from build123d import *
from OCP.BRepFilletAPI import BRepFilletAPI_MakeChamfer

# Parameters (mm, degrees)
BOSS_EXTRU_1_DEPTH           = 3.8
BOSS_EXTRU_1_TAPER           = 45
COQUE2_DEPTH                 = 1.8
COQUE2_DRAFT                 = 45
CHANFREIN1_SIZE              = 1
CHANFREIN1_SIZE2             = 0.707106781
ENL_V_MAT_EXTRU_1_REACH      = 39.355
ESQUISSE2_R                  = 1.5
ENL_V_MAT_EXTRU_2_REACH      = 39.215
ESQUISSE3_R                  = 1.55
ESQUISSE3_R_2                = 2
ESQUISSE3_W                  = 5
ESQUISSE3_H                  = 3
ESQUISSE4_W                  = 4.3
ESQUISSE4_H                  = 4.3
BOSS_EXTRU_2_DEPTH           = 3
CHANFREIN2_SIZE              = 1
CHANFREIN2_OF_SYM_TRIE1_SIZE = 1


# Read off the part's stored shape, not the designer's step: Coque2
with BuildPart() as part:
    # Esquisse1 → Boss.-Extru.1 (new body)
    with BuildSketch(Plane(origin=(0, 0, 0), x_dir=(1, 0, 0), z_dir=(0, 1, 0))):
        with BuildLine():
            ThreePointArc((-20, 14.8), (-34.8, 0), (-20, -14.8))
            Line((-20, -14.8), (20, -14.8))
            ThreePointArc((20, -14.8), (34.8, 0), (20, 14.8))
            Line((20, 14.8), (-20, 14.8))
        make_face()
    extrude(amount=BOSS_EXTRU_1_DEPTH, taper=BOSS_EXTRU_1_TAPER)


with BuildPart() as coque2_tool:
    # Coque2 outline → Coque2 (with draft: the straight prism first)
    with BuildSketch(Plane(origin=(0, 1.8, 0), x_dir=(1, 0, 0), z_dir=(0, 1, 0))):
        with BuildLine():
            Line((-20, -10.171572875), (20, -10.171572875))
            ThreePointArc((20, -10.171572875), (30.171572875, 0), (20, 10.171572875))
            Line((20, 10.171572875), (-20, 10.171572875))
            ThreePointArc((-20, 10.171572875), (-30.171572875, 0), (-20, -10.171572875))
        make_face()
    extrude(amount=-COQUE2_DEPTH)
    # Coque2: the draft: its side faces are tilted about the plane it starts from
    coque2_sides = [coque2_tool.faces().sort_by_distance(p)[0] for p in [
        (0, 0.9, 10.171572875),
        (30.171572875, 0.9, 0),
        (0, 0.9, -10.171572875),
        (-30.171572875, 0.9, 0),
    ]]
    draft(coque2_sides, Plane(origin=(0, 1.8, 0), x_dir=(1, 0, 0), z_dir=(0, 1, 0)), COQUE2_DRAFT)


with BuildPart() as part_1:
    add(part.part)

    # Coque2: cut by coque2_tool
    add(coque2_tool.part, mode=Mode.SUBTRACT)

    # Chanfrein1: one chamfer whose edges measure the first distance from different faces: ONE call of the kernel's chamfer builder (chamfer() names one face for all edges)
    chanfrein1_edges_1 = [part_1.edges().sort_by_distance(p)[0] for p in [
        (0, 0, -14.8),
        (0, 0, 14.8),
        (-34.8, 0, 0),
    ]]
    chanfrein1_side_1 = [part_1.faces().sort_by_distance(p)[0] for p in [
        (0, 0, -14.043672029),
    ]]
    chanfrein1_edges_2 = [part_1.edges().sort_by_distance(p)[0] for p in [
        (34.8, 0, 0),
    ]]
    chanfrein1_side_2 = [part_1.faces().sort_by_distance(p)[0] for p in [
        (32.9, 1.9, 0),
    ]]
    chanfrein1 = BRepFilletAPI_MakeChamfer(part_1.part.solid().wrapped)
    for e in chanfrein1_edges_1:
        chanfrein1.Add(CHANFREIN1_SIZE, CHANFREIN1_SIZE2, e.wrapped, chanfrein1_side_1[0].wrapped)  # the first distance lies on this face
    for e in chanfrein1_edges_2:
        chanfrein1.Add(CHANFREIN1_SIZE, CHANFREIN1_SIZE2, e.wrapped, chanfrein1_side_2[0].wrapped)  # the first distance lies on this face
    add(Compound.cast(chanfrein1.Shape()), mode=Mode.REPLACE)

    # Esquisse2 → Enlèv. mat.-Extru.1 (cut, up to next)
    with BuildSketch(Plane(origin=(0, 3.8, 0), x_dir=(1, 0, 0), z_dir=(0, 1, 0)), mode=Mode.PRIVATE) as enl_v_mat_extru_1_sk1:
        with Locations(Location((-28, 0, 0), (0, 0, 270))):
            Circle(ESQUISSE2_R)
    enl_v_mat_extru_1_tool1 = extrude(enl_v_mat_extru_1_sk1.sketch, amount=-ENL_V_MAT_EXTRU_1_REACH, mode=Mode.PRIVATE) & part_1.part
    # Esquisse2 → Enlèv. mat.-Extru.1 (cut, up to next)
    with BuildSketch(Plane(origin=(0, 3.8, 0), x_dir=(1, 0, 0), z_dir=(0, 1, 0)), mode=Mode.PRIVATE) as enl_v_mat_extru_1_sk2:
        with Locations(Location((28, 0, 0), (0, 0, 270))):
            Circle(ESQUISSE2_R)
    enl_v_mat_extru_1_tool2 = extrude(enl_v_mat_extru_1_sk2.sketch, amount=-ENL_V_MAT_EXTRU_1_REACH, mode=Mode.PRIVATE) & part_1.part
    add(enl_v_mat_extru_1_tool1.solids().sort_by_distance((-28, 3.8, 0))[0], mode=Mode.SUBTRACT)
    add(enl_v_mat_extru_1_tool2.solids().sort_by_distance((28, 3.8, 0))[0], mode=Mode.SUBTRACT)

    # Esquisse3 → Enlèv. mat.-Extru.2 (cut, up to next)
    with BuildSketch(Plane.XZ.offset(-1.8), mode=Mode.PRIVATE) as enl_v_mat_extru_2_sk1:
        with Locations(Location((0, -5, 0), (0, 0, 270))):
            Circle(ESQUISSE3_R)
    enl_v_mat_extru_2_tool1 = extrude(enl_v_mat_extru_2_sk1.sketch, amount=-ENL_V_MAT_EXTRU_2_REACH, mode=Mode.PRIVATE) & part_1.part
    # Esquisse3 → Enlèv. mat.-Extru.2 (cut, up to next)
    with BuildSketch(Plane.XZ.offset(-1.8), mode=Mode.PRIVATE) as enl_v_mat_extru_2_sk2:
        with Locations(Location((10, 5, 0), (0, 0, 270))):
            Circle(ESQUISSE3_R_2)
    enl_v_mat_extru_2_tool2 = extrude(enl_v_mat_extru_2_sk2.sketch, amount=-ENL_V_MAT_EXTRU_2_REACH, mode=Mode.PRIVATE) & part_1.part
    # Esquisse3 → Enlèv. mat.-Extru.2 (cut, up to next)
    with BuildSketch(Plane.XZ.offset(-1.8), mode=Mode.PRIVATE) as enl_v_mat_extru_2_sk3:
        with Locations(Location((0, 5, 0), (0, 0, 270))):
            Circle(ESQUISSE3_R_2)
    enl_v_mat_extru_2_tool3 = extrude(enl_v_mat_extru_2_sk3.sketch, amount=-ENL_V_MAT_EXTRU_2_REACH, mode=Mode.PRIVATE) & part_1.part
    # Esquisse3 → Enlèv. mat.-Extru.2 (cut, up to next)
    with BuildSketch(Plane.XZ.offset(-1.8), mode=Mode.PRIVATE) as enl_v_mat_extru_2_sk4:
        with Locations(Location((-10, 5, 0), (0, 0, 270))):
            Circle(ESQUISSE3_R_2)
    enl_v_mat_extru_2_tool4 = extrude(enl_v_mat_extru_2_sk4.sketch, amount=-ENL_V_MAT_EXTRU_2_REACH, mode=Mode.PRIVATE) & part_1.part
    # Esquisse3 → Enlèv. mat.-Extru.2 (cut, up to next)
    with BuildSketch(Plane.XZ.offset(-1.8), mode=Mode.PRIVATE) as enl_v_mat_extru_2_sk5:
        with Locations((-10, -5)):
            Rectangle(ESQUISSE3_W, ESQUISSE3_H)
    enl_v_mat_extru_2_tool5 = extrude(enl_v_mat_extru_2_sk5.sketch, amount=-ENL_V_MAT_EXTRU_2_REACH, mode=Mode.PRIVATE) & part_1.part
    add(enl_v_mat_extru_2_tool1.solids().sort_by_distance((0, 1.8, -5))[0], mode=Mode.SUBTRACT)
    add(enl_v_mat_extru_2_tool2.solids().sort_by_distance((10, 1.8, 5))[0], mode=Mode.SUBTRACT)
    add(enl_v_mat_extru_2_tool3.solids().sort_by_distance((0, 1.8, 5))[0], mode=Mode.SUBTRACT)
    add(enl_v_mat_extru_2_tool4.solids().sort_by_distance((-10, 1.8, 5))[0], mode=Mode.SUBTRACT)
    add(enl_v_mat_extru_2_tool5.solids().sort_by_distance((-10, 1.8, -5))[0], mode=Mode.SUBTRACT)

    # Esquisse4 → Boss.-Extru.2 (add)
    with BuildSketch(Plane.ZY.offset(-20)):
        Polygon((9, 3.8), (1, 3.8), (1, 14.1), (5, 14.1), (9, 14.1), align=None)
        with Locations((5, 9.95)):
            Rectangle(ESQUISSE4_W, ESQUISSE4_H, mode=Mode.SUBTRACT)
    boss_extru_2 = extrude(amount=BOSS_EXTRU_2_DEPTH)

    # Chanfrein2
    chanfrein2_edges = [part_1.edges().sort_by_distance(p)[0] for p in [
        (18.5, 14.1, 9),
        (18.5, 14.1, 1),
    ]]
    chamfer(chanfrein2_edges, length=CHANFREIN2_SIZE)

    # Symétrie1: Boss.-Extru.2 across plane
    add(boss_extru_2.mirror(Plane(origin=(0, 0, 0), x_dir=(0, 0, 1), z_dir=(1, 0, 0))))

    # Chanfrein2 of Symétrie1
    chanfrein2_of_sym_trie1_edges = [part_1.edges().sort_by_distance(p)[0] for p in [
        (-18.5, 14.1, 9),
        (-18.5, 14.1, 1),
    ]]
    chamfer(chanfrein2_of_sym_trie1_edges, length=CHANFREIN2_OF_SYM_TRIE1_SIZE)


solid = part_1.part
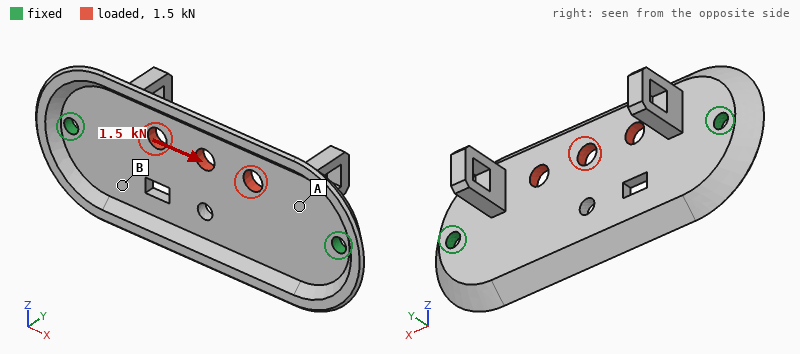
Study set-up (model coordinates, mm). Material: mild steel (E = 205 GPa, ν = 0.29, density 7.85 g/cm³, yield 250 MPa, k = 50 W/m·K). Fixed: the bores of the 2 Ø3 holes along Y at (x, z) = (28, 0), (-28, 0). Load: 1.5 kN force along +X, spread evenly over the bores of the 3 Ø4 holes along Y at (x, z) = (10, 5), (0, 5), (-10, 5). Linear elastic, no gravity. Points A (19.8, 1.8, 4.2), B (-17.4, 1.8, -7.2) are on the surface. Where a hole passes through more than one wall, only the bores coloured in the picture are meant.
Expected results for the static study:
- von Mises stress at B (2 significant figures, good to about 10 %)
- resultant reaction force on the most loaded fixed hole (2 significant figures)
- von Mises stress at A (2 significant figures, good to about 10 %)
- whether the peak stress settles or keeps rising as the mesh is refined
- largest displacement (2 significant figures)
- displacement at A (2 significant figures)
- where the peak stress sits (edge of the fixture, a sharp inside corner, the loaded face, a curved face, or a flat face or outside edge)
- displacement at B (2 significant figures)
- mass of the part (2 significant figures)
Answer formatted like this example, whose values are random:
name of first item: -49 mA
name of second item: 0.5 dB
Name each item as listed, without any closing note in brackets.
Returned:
von Mises stress at B: 7.9 MPa
resultant reaction force on the most loaded fixed hole: 770 N
von Mises stress at A: 29 MPa
whether the peak stress settles or keeps rising as the mesh is refined: keeps rising
largest displacement: 3.6 µm
displacement at A: 1.6 µm
where the peak stress sits: edge of the fixture
displacement at B: 1.4 µm
mass of the part: 30 g
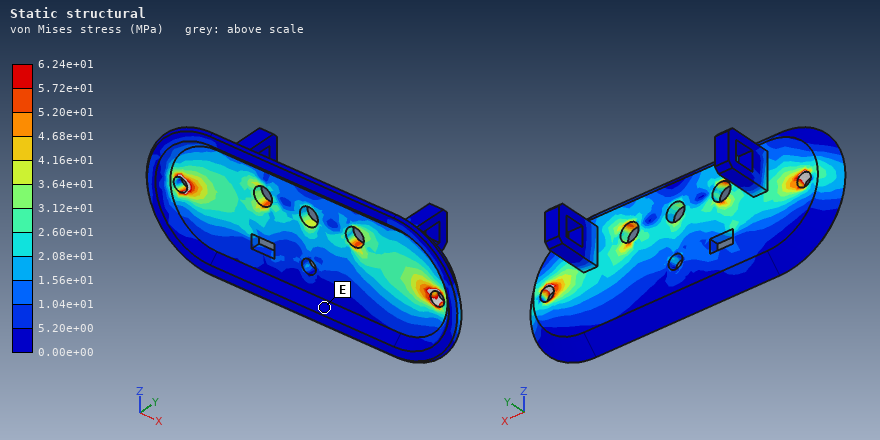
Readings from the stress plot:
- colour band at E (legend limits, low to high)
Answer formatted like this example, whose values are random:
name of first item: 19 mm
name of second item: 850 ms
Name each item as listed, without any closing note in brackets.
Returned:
colour band at E: 0.00e+00 to 5.20e+00 MPa
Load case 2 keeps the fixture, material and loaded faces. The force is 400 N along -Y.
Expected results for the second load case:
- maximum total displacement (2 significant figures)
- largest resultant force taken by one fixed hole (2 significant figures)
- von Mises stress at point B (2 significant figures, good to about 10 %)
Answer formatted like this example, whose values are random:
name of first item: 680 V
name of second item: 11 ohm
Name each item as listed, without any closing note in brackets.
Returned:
maximum total displacement: 98 µm
largest resultant force taken by one fixed hole: 280 N
von Mises stress at point B: 56 MPa
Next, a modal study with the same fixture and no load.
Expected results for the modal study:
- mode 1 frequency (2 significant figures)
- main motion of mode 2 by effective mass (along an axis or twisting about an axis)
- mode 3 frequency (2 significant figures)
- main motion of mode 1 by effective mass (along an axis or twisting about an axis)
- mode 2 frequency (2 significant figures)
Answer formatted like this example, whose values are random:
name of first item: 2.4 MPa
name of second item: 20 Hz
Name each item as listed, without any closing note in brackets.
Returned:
mode 1 frequency: 3500 Hz
main motion of mode 2 by effective mass: twisting about X
mode 3 frequency: 7800 Hz
main motion of mode 1 by effective mass: along Y
mode 2 frequency: 4000 Hz
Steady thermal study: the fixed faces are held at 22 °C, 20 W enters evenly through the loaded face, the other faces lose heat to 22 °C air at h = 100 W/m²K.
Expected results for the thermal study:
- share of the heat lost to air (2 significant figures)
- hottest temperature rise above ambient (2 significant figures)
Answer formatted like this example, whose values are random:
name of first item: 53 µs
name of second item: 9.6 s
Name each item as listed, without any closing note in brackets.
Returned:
share of the heat lost to air: 59 %
hottest temperature rise above ambient: 69 K
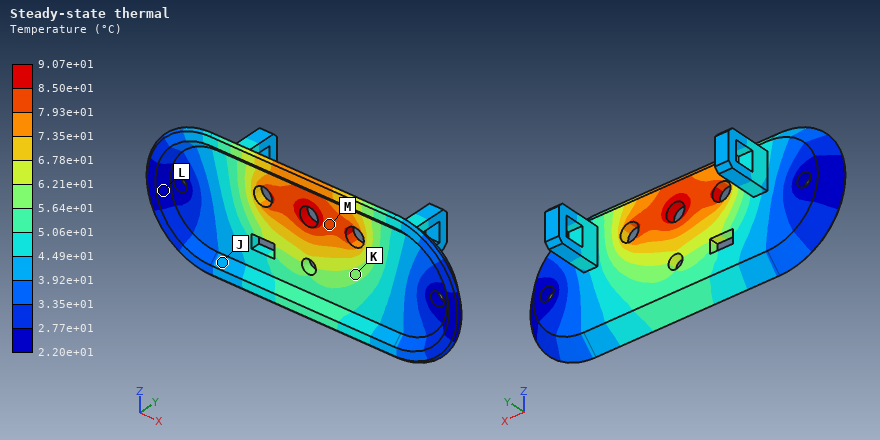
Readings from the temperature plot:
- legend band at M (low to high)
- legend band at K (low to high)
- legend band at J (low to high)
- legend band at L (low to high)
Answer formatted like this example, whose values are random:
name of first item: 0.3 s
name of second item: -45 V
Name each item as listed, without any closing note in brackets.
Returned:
legend band at M: 7.93e+01 to 8.50e+01 °C
legend band at K: 5.64e+01 to 6.21e+01 °C
legend band at J: 3.92e+01 to 4.49e+01 °C
legend band at L: 2.20e+01 to 2.77e+01 °C
